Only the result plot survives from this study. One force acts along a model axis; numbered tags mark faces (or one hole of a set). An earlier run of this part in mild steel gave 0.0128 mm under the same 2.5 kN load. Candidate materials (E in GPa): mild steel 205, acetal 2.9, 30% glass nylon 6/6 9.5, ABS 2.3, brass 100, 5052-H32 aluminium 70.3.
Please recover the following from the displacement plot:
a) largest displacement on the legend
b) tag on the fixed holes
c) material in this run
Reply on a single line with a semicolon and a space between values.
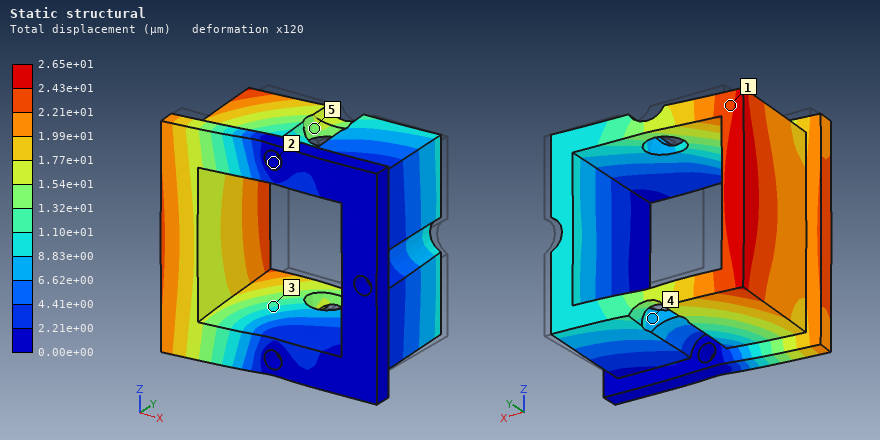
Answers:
2.65e+01 µm; 2; brass
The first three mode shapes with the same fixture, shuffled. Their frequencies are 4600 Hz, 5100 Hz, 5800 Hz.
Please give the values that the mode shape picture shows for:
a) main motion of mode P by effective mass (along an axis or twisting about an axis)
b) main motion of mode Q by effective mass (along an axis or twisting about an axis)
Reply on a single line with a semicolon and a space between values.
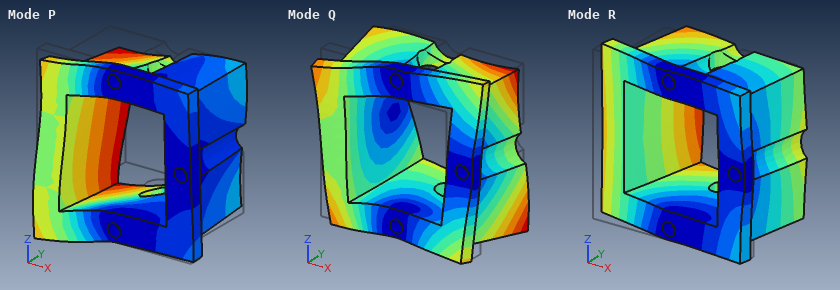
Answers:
along Z; along Z
